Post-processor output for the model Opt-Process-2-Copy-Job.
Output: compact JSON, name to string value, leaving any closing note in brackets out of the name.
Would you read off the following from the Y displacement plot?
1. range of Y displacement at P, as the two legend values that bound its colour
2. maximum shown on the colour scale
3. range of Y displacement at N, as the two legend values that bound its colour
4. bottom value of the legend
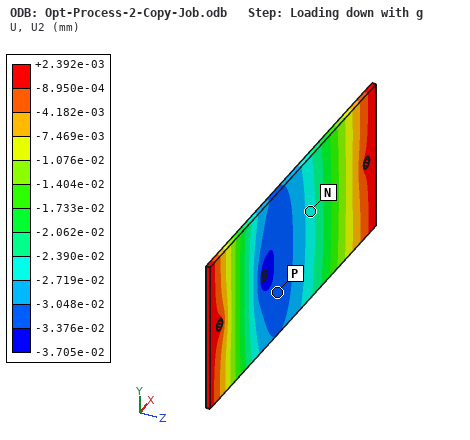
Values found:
{"range of Y displacement at P, as the two legend values that bound its colour": "-3.376e-02 to -3.048e-02 mm", "maximum shown on the colour scale": "+2.392e-03 mm", "range of Y displacement at N, as the two legend values that bound its colour": "-2.719e-02 to -2.390e-02 mm", "bottom value of the legend": "-3.705e-02 mm"}
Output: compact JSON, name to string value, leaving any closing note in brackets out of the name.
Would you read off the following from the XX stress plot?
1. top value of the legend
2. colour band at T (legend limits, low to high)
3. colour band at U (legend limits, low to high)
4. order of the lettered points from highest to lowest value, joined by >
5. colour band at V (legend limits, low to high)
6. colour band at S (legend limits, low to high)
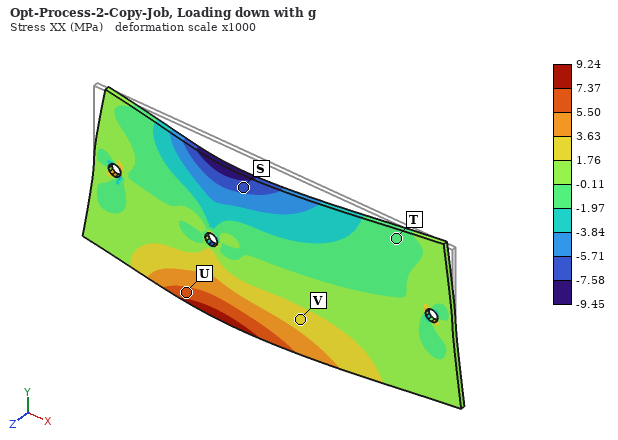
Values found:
{"top value of the legend": "9.24 MPa", "colour band at T": "-1.97 to -0.11 MPa", "colour band at U": "5.50 to 7.37 MPa", "order of the lettered points from highest to lowest value, joined by >": "U > V > T > S", "colour band at V": "1.76 to 3.63 MPa", "colour band at S": "-7.58 to -5.71 MPa"}
